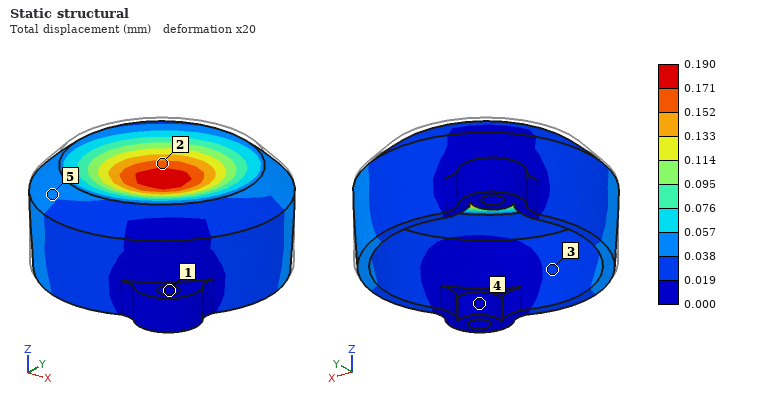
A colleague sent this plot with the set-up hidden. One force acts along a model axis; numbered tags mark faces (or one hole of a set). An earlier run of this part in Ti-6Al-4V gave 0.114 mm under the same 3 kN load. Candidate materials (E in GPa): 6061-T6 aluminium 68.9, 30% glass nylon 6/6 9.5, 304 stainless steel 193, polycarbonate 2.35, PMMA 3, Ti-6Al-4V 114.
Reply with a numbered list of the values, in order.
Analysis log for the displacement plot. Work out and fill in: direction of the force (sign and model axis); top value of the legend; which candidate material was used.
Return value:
1. -Z
2. 0.190 mm
3. 6061-T6 aluminium
